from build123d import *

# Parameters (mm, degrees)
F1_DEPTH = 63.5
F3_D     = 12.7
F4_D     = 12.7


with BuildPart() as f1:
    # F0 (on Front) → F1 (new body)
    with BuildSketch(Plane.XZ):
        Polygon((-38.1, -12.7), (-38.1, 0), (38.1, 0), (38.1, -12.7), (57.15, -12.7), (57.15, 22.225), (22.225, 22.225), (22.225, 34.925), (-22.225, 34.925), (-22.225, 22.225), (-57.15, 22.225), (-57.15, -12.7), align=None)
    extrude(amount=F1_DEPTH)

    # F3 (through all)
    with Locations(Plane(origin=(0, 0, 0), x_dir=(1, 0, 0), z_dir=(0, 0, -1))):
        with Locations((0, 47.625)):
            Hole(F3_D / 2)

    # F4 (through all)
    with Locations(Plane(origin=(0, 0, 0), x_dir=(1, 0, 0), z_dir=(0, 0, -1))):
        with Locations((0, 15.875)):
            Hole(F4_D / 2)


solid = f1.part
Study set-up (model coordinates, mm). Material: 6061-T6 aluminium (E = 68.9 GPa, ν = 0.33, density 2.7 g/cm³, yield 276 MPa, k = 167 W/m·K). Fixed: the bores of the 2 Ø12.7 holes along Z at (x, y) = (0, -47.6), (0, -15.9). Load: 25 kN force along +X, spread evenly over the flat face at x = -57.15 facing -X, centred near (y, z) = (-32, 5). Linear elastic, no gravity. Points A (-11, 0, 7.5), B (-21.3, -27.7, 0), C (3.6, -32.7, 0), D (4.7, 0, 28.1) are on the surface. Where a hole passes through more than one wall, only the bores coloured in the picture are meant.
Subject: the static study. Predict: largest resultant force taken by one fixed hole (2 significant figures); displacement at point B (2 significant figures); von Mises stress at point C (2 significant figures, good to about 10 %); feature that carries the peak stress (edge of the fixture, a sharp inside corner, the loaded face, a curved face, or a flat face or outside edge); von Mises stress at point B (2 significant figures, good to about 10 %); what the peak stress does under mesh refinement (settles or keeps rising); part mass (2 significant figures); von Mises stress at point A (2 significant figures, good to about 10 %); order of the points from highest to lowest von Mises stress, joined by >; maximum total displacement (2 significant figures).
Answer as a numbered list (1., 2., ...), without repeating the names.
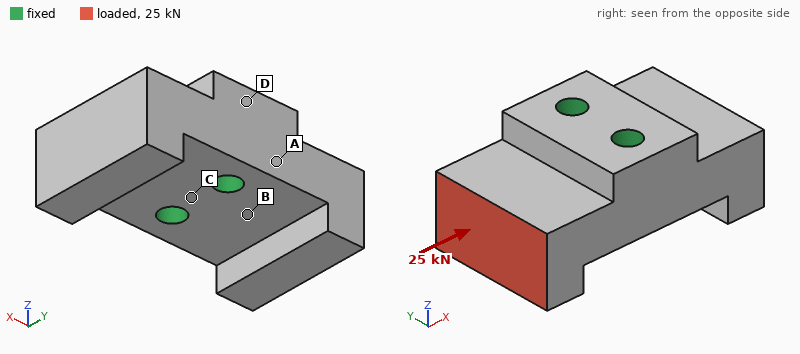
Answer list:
1. 13 kN
2. 13 µm
3. 12 MPa
4. edge of the fixture
5. 42 MPa
6. keeps rising
7. 590 g
8. 19 MPa
9. B > A > C > D
10. 71 µm
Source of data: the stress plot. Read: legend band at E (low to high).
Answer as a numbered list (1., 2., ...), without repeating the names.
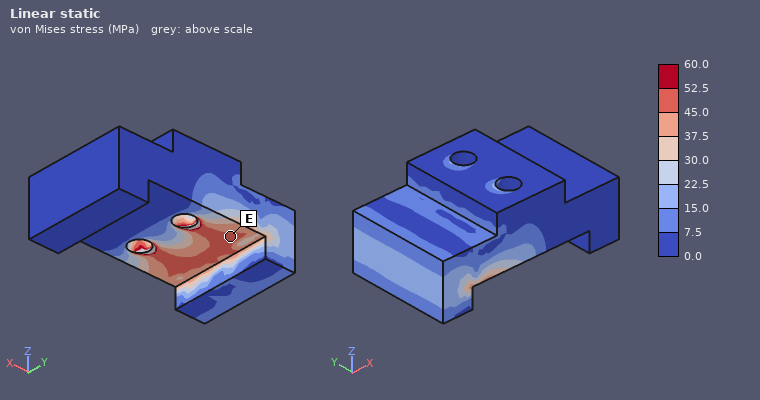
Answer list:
1. 45.0 to 52.5 MPa
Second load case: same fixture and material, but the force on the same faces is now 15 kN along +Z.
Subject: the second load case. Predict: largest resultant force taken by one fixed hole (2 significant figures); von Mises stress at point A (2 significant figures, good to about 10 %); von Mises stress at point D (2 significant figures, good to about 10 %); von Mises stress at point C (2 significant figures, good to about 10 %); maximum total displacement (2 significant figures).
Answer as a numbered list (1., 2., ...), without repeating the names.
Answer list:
1. 7.5 kN
2. 28 MPa
3. 13 MPa
4. 22 MPa
5. 0.17 mm
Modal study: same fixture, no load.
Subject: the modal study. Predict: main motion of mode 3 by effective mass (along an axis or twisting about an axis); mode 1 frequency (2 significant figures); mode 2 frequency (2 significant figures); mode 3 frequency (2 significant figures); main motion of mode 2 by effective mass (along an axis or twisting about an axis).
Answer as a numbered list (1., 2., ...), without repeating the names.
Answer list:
1. twisting about Z
2. 5600 Hz
3. 5800 Hz
4. 8100 Hz
5. along Z
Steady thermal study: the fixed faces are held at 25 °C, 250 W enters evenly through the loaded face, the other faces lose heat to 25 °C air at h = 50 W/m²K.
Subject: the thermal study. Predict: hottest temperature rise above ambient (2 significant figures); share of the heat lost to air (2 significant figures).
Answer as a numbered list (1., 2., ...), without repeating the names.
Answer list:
1. 49 K
2. 5.7 %
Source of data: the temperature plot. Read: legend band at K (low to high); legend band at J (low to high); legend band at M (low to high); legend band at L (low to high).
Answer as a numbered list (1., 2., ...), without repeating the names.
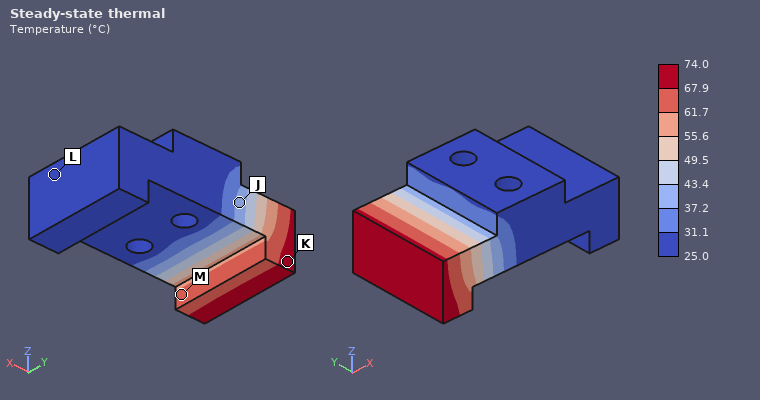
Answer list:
1. 67.9 to 74.0 °C
2. 37.2 to 43.4 °C
3. 61.7 to 67.9 °C
4. 25.0 to 31.1 °C
